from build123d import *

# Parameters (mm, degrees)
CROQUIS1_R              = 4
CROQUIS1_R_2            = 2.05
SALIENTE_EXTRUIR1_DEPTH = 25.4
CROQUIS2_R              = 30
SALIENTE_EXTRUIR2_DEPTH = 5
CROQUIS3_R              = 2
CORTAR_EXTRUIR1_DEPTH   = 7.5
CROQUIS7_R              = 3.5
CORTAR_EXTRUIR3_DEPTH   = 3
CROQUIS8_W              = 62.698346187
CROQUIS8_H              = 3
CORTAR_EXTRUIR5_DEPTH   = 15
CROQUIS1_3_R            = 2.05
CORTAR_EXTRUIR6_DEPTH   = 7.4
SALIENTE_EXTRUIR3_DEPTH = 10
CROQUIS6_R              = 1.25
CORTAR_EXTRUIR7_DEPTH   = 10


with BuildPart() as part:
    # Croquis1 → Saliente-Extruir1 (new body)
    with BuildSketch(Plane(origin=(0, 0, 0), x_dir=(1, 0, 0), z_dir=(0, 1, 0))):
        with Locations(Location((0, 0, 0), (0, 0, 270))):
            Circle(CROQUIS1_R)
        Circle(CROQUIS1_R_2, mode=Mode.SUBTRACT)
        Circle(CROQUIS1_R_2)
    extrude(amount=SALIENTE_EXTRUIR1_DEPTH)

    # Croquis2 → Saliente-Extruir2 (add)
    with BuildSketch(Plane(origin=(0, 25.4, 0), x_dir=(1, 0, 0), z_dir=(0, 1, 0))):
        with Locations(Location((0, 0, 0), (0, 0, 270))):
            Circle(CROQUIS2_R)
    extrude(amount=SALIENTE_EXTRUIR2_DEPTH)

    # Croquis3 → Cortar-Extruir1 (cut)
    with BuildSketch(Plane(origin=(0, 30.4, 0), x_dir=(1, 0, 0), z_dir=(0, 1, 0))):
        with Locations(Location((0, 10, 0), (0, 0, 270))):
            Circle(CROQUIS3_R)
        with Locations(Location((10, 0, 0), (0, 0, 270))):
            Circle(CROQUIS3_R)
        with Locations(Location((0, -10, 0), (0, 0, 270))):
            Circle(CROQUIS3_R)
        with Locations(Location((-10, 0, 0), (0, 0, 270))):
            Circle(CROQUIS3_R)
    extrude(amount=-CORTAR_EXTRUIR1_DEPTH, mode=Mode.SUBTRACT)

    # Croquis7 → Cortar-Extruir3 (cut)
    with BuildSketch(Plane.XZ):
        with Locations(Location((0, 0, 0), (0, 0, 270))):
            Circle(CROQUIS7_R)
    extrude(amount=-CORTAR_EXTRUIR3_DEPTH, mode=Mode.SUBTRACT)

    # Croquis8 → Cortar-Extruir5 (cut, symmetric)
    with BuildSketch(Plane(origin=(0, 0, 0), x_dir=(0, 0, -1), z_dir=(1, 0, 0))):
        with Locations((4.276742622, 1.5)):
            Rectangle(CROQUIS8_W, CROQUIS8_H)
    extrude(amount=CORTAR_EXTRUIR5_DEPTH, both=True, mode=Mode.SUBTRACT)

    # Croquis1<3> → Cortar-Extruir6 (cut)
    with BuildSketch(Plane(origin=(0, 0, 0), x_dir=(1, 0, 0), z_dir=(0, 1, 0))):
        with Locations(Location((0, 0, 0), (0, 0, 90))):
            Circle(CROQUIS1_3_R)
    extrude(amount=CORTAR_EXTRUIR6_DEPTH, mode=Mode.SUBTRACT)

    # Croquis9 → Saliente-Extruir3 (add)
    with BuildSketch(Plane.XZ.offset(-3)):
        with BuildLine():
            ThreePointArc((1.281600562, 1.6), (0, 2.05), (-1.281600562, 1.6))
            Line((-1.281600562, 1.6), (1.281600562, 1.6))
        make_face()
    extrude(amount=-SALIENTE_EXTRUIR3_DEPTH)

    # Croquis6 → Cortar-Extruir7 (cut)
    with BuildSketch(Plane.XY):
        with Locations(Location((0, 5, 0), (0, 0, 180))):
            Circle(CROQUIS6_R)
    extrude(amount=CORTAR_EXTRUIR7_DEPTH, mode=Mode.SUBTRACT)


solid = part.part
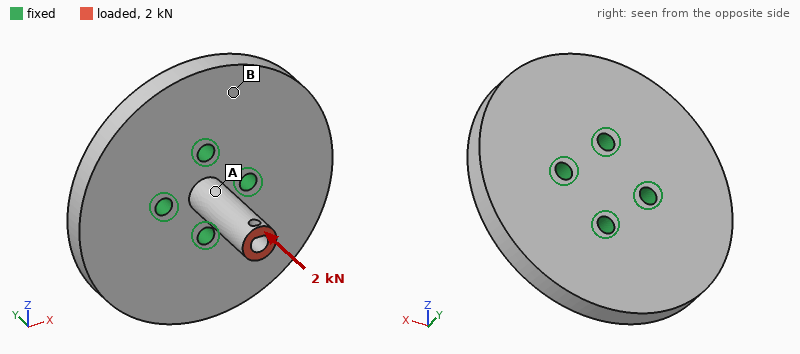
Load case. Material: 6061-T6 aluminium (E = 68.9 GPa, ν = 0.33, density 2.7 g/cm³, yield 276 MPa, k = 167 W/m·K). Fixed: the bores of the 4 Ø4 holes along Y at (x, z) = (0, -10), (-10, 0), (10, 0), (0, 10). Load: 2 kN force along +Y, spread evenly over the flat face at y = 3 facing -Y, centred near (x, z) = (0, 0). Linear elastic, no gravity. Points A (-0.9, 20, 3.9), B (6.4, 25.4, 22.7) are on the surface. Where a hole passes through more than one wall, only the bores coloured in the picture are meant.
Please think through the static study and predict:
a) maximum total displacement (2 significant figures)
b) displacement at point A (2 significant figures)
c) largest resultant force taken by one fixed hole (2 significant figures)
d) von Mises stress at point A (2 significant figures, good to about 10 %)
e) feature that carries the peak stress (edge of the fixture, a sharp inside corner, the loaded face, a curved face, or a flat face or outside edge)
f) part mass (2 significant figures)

29 µm
8.2 µm
520 N
40 MPa
a curved face
40 g
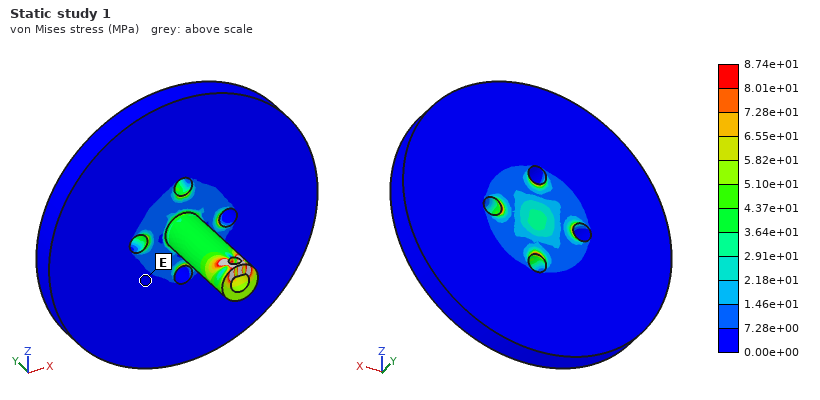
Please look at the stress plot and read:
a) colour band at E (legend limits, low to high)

0.00e+00 to 7.28e+00 MPa
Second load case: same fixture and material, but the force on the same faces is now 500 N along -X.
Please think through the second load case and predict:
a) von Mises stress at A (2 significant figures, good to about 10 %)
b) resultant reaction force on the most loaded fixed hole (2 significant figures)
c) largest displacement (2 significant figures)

41 MPa
750 N
0.20 mm
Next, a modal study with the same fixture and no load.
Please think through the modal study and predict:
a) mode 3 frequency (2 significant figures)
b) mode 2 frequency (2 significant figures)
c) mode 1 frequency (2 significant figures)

9300 Hz
9000 Hz
8900 Hz
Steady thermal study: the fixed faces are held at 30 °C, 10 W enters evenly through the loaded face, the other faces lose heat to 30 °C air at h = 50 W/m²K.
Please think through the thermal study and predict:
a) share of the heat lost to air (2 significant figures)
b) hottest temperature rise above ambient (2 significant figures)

6.3 %
34 K
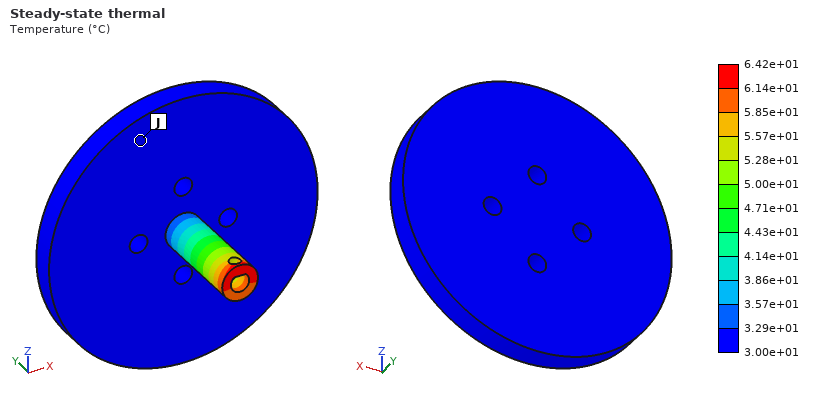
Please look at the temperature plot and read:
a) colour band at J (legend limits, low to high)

3.00e+01 to 3.29e+01 °C
